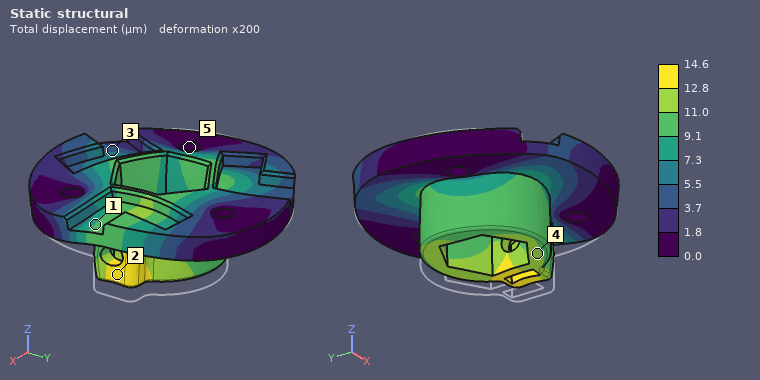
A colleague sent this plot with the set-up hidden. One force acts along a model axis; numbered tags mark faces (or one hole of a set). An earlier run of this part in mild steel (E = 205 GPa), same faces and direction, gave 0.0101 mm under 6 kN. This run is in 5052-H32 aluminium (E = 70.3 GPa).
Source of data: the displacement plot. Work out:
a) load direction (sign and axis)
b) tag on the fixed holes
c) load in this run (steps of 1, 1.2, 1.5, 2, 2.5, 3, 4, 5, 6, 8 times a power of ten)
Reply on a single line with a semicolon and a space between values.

+Z; 5; 3 kN
